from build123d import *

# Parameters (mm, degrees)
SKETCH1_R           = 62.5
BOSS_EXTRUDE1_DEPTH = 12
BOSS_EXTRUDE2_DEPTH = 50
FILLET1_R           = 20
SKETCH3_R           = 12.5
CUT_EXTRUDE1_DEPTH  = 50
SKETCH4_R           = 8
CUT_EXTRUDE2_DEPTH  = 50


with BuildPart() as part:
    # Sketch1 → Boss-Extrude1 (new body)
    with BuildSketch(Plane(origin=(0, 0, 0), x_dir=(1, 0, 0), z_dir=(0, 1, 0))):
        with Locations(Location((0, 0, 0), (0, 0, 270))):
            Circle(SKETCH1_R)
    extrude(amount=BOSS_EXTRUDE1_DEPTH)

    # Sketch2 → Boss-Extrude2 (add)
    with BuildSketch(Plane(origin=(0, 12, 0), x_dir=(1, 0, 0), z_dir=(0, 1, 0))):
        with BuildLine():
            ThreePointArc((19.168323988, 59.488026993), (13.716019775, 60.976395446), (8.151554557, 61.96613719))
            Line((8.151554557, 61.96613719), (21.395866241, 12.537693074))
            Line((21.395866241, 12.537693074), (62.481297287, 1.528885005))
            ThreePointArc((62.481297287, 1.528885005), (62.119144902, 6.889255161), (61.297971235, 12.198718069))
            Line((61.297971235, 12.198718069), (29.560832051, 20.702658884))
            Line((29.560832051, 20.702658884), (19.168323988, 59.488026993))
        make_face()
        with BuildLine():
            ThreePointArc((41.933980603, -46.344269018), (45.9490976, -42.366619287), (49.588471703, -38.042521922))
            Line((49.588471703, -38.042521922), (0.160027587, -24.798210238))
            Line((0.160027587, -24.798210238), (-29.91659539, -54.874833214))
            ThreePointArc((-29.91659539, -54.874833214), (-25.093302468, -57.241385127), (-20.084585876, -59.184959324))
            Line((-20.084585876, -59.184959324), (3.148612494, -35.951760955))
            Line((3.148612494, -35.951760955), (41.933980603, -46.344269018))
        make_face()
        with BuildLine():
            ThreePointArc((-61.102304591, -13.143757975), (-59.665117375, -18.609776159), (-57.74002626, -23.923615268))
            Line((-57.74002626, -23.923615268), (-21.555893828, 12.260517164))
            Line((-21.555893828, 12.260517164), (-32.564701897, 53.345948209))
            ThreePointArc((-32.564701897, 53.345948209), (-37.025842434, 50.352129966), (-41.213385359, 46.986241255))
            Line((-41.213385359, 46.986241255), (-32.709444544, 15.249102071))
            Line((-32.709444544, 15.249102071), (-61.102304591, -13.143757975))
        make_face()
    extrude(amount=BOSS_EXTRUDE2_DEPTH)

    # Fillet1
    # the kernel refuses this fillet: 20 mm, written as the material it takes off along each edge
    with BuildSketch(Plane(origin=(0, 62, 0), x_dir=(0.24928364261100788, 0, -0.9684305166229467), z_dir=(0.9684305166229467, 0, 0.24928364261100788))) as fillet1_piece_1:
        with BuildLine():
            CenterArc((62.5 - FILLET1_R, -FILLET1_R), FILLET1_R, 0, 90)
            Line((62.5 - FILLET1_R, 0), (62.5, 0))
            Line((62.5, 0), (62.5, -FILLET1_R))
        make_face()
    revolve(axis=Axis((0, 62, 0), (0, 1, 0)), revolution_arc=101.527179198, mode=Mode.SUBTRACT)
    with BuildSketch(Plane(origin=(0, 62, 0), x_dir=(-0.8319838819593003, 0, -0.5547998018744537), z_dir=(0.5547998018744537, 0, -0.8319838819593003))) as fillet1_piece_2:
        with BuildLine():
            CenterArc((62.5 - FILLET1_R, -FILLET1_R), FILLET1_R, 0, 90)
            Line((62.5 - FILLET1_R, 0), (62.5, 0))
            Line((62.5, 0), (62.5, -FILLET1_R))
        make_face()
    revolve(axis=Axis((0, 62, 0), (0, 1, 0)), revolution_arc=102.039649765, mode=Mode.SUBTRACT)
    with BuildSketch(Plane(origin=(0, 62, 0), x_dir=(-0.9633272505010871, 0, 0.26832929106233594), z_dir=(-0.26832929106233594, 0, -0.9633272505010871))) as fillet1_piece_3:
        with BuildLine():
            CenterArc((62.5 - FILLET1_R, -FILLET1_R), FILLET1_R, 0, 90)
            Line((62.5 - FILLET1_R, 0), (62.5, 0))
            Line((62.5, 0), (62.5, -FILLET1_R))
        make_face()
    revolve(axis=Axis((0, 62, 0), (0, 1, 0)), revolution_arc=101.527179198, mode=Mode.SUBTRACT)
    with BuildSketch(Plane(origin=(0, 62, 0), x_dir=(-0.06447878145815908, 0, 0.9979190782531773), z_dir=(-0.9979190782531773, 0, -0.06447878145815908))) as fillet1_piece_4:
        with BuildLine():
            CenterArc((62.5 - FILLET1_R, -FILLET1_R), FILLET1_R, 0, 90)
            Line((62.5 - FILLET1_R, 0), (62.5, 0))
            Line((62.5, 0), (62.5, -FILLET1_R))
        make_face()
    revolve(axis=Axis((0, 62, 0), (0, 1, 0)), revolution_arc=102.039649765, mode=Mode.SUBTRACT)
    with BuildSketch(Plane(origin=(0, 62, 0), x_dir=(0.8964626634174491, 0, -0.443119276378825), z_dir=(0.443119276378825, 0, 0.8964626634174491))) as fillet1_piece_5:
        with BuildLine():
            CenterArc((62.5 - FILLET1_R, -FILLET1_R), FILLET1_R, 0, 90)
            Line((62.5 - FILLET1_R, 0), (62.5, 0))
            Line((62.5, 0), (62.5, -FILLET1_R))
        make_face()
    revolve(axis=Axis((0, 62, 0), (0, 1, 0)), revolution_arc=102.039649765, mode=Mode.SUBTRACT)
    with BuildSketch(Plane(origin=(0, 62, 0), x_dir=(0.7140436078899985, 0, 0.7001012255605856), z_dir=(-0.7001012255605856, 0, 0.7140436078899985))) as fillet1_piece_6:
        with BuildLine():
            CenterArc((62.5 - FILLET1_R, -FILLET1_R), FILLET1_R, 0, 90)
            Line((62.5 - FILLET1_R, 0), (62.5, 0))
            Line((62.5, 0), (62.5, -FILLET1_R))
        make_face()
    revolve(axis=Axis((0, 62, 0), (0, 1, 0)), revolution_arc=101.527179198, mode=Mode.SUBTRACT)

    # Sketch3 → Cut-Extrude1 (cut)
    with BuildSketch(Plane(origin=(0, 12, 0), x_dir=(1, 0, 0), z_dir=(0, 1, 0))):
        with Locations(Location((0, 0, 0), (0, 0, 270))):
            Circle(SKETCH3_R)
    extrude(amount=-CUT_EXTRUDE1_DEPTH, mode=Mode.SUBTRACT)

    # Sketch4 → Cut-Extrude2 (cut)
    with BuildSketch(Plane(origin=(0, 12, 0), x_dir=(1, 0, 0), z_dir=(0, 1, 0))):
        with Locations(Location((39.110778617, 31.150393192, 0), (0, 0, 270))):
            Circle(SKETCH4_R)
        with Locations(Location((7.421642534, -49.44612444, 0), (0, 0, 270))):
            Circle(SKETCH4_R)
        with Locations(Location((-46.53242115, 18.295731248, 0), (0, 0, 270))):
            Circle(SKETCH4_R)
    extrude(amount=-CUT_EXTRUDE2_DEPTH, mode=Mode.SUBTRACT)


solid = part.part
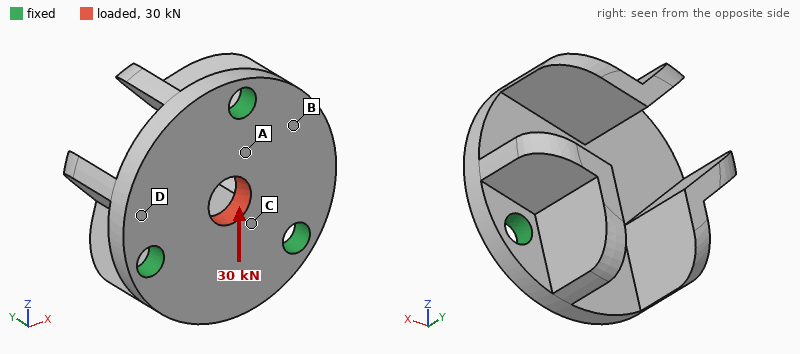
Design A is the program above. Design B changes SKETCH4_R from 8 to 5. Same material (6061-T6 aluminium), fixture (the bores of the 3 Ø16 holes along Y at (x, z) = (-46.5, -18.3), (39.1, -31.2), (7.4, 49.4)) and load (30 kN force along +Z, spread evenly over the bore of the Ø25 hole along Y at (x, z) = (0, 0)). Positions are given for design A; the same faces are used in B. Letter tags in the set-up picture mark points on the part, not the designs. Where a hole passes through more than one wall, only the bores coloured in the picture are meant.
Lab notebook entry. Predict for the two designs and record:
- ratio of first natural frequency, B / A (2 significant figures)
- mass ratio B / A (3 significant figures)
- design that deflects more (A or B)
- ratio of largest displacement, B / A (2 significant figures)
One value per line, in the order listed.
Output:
0.90
1.02
B
1.1
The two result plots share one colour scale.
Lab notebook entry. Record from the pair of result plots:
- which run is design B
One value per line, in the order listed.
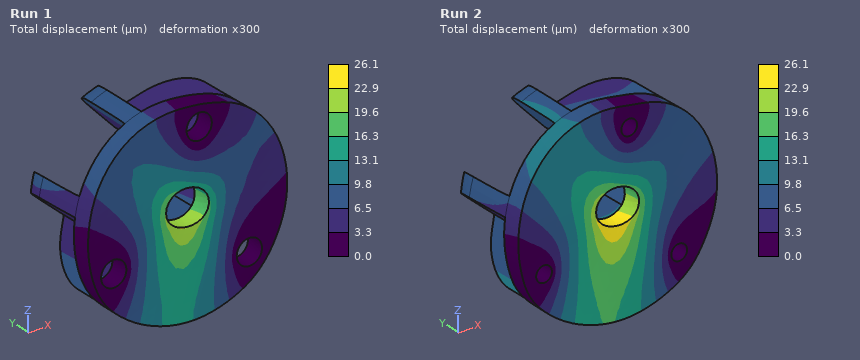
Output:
Run 2
